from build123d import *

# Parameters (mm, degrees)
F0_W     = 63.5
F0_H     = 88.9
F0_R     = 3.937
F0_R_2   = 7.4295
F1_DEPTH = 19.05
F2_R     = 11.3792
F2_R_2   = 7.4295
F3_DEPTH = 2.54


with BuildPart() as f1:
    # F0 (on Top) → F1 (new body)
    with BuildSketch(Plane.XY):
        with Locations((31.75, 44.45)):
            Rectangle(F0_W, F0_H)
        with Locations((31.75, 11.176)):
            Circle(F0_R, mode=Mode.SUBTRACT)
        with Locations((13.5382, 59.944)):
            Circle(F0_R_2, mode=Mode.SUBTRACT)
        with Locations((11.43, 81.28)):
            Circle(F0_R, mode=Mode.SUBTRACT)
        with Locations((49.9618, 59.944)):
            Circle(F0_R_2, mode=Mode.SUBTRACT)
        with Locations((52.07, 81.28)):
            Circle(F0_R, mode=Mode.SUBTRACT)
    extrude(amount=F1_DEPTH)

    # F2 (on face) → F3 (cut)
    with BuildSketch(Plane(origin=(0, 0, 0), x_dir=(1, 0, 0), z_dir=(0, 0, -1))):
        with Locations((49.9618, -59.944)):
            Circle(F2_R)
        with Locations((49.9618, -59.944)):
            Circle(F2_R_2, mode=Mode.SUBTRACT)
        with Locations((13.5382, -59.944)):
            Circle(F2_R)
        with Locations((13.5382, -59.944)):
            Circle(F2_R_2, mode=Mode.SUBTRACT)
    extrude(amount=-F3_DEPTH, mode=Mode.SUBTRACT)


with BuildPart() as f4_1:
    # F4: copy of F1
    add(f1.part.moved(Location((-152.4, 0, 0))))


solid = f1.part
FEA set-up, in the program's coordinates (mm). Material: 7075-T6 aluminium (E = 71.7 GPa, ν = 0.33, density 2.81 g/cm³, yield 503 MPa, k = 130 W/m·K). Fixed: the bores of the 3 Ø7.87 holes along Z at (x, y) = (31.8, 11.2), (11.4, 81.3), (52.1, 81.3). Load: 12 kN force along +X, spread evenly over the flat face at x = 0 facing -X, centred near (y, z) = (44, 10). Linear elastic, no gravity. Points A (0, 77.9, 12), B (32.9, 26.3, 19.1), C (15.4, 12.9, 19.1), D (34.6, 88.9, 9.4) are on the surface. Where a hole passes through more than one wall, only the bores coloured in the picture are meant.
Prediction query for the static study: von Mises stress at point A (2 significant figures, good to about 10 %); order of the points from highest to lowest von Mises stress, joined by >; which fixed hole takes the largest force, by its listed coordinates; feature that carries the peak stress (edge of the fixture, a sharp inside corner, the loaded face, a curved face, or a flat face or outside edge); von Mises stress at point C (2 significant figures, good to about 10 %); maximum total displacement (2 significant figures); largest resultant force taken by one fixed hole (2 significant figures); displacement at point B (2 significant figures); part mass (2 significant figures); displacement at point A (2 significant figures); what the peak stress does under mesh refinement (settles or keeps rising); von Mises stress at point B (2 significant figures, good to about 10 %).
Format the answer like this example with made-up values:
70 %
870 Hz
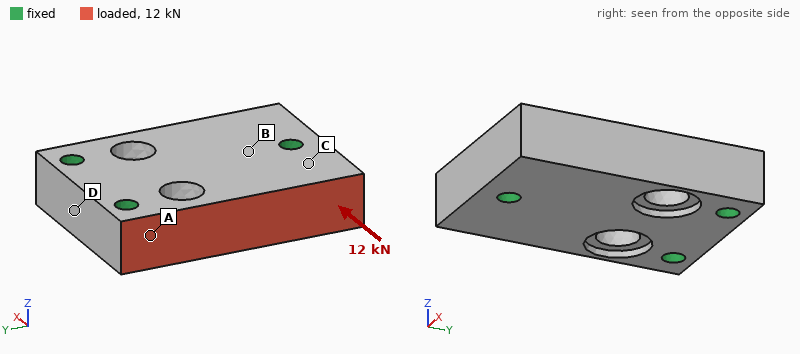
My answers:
13 MPa
A > C > B > D
(31.8, 11.2)
edge of the fixture
9.6 MPa
11 µm
6.1 kN
3.1 µm
270 g
2.0 µm
keeps rising
5.3 MPa
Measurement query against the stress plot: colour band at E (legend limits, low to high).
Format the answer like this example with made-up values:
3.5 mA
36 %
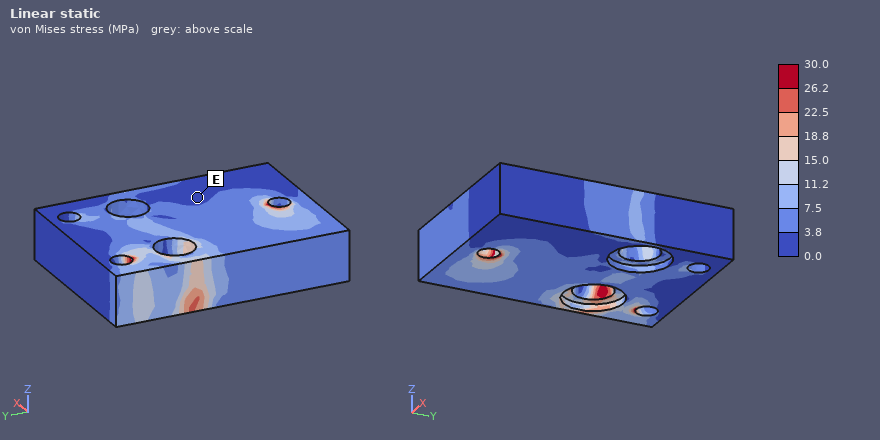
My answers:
0.0 to 3.8 MPa
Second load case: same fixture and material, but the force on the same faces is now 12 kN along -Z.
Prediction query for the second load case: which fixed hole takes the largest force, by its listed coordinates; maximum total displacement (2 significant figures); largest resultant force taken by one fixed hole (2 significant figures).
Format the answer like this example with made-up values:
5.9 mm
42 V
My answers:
(11.4, 81.3)
63 µm
7.1 kN
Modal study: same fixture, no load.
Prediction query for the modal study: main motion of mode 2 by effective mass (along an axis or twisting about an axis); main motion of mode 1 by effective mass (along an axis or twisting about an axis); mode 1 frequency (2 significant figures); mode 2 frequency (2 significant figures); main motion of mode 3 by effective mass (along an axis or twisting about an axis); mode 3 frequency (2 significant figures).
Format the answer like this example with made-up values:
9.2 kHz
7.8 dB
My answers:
along Z
twisting about Y
10 kHz
11 kHz
along X
15 kHz
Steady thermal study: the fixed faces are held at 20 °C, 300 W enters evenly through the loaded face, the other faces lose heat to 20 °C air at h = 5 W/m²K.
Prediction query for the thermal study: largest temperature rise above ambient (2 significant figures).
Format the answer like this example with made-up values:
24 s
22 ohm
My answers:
55 K
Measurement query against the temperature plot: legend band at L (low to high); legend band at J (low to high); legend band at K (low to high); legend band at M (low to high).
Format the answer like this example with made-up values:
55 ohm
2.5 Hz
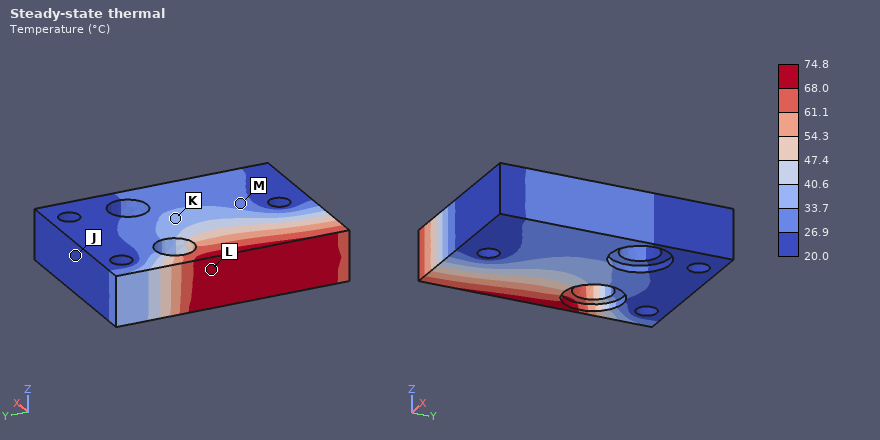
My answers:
68.0 to 74.8 °C
20.0 to 26.9 °C
33.7 to 40.6 °C
26.9 to 33.7 °C
